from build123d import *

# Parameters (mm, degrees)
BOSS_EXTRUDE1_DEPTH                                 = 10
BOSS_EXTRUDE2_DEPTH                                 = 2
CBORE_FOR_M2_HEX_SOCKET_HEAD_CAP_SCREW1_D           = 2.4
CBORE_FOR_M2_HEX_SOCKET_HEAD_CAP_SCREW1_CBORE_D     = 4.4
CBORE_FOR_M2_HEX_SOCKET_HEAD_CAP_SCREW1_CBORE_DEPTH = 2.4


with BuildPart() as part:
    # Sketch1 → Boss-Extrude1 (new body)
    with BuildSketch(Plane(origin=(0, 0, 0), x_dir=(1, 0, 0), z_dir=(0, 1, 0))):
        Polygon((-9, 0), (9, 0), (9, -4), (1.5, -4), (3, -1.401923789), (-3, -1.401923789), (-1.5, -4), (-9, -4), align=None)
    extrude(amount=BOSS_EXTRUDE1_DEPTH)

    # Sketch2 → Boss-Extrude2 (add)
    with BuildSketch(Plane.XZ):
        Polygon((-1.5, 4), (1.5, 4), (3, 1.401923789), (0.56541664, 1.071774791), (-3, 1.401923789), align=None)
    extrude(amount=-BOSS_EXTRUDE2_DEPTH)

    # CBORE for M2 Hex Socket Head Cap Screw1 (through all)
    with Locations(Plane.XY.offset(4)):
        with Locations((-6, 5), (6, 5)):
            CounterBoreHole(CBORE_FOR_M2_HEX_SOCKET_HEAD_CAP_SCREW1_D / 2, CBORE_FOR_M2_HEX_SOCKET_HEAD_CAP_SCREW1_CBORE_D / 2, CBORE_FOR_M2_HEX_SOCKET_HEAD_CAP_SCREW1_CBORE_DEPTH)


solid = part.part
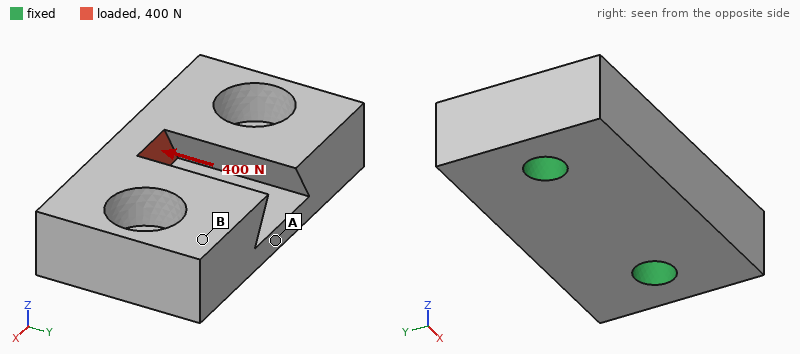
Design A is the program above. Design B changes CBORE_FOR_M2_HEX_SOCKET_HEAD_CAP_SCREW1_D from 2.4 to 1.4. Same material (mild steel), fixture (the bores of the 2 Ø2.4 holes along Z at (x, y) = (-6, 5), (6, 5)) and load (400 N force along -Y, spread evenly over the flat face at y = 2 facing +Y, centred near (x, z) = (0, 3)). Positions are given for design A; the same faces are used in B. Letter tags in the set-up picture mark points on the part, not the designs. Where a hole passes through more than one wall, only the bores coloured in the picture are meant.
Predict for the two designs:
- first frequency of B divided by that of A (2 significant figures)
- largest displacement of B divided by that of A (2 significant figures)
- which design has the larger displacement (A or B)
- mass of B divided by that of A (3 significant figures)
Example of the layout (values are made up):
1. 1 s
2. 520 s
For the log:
1. 0.69
2. 1.5
3. B
4. 1.02
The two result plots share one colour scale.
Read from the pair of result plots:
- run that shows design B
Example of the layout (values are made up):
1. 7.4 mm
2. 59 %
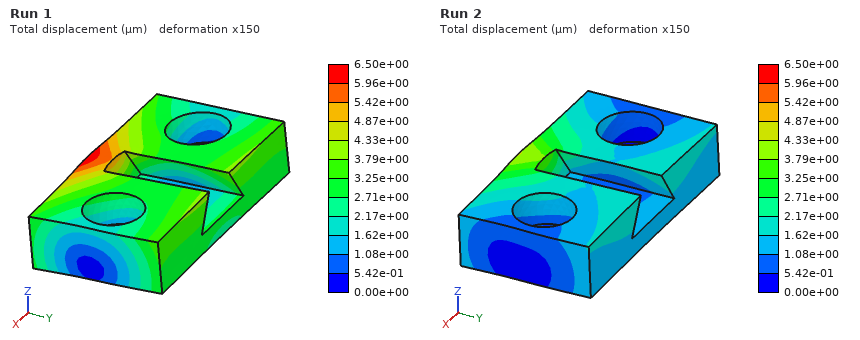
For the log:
1. Run 1
